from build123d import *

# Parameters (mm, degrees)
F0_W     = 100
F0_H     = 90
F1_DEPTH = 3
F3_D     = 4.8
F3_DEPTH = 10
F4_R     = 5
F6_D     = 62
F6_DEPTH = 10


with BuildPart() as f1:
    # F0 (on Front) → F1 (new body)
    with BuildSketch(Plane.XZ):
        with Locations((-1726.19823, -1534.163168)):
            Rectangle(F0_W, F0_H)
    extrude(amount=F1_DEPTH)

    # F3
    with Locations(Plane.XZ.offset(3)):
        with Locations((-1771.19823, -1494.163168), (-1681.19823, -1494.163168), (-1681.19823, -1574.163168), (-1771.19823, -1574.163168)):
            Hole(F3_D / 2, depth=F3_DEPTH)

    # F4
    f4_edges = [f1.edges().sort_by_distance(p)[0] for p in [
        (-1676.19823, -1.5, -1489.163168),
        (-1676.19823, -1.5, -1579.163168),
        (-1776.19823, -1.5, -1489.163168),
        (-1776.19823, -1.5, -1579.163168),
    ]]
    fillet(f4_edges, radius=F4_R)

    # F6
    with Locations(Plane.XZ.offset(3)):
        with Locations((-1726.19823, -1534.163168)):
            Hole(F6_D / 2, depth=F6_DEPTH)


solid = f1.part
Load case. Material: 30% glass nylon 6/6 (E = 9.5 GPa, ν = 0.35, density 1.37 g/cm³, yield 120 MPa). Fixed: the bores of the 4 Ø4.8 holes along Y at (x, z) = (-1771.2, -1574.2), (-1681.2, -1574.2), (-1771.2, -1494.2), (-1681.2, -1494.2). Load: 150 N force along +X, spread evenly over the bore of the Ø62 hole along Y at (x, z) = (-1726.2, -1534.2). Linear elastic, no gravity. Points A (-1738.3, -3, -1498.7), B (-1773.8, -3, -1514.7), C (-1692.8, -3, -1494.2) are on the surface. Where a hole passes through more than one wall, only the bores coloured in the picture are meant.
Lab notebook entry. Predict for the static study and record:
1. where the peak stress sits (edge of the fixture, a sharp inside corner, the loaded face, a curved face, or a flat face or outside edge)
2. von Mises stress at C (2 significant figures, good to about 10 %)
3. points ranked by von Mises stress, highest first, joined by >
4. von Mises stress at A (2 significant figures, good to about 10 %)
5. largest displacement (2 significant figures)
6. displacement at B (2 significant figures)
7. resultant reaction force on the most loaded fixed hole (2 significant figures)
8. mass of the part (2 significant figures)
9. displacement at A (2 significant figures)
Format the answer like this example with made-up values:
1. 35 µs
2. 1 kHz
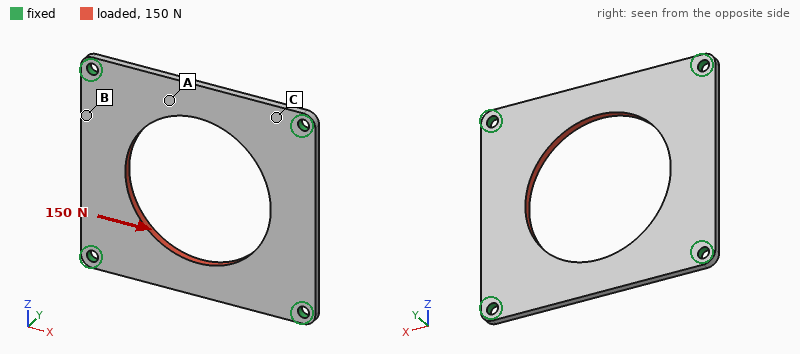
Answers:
1. edge of the fixture
2. 0.75 MPa
3. C > A > B
4. 0.51 MPa
5. 6.2 µm
6. 4.1 µm
7. 40 N
8. 24 g
9. 2.7 µm
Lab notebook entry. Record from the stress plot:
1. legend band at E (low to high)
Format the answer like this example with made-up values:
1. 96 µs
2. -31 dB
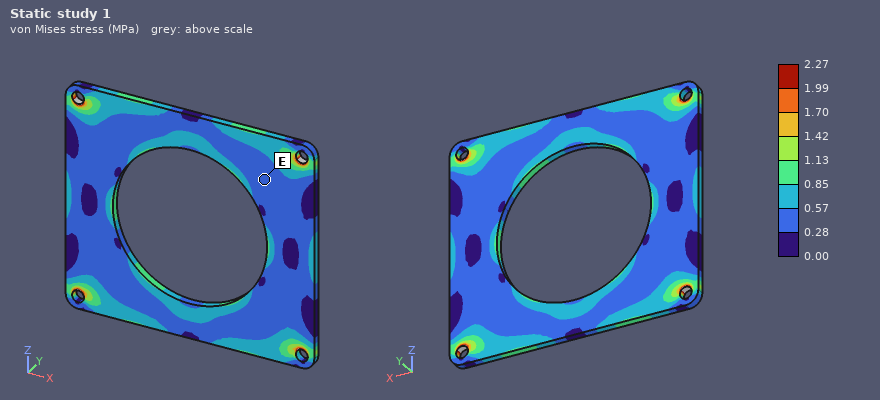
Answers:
1. 0.28 to 0.57 MPa
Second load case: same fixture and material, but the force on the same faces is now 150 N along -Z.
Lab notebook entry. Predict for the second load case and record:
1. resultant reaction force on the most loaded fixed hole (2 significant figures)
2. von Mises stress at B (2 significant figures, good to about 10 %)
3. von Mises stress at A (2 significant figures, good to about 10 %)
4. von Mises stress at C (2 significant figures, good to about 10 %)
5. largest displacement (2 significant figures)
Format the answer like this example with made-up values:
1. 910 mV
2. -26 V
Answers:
1. 40 N
2. 0.81 MPa
3. 0.50 MPa
4. 0.36 MPa
5. 8.2 µm
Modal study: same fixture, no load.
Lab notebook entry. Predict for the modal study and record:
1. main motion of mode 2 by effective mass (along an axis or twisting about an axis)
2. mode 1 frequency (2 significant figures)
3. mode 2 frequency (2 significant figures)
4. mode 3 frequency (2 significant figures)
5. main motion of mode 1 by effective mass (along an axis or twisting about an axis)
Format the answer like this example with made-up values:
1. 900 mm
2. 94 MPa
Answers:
1. twisting about X
2. 990 Hz
3. 1200 Hz
4. 1300 Hz
5. along Y
